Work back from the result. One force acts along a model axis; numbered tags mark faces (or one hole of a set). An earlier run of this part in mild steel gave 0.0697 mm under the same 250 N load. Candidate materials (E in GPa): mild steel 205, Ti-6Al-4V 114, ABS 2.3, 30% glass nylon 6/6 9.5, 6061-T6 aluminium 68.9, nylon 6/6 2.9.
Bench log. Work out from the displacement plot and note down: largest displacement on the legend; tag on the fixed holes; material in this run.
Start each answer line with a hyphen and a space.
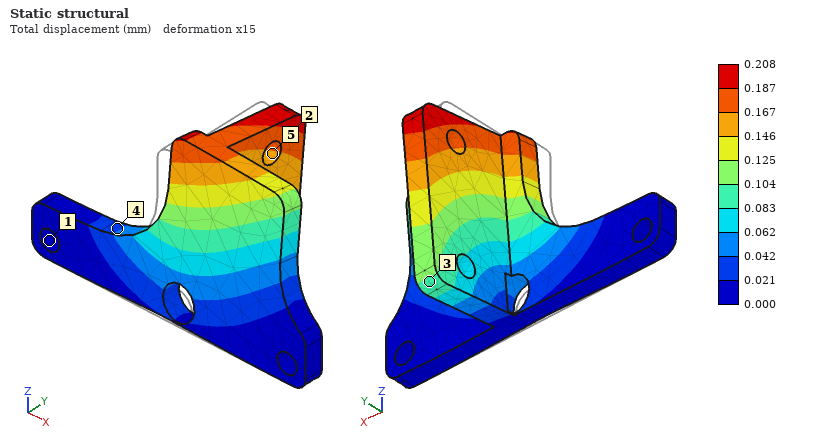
- 0.208 mm
- 1
- 6061-T6 aluminium
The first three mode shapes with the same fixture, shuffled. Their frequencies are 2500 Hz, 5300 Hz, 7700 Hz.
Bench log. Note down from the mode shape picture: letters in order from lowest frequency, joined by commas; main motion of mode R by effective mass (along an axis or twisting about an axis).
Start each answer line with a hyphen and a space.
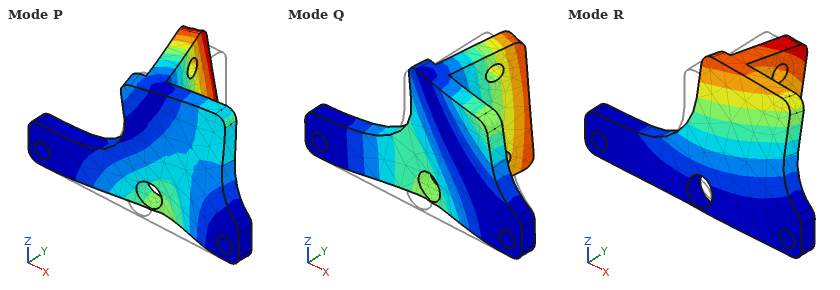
- R, Q, P
- along Y
